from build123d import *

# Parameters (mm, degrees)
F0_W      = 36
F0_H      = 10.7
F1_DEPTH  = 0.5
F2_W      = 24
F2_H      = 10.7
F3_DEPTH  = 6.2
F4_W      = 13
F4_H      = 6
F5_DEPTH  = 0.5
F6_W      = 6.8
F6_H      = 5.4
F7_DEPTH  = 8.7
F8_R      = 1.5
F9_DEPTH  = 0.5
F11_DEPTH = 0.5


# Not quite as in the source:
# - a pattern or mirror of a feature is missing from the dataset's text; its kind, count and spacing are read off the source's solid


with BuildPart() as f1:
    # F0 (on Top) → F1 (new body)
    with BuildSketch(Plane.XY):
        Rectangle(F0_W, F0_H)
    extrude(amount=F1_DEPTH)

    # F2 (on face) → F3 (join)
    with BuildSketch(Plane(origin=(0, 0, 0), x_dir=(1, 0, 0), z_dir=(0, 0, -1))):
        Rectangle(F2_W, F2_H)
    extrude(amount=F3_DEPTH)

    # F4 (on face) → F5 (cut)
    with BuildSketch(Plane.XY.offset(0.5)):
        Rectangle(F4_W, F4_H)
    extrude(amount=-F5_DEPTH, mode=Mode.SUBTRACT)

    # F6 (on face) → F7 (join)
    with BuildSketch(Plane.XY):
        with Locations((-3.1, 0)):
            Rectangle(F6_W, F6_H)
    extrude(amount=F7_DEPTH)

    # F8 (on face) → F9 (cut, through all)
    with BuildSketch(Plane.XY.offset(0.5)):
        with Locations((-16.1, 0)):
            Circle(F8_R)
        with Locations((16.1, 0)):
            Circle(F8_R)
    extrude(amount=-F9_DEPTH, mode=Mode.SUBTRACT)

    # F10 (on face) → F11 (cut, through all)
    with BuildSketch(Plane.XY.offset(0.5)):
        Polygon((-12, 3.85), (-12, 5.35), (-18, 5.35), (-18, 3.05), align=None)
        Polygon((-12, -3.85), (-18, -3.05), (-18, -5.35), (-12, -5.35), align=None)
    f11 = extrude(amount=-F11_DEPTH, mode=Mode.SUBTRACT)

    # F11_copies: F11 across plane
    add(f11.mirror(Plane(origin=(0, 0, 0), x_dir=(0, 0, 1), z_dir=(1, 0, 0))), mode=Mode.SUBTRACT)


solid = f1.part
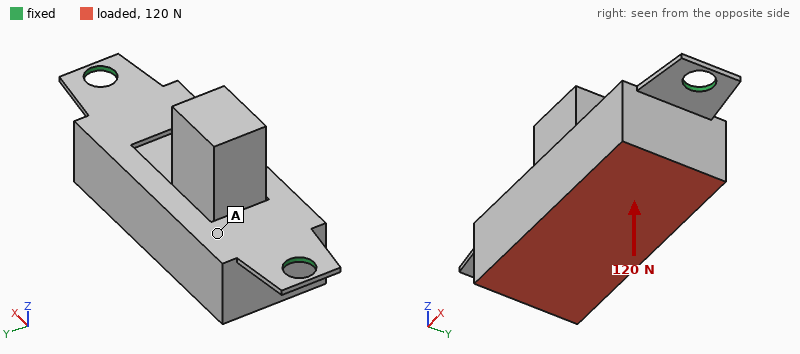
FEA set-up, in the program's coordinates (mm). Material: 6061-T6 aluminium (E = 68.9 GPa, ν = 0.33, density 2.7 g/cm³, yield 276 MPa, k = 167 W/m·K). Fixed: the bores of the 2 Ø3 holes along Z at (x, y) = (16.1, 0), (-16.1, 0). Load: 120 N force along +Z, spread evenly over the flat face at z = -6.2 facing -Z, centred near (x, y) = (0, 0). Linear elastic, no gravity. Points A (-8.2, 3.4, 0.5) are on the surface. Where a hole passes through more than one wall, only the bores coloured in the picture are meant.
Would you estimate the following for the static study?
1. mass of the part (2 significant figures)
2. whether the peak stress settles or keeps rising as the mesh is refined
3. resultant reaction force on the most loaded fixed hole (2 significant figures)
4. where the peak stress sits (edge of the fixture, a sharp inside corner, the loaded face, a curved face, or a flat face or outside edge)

5.5 g
keeps rising
76 N
edge of the fixture
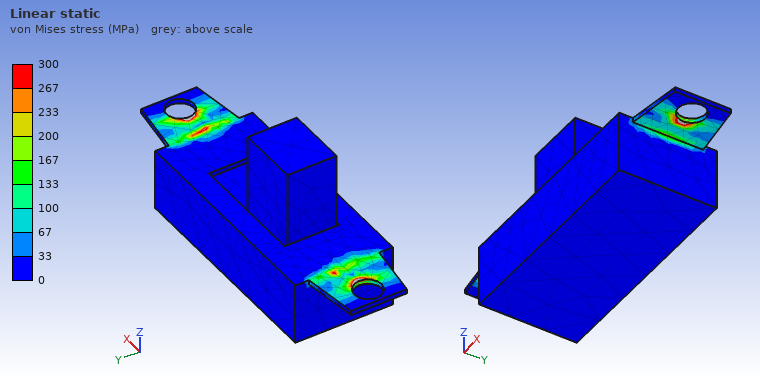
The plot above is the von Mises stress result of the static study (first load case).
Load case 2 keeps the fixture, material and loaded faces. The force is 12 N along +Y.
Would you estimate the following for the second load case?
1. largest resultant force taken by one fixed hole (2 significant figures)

6.0 N
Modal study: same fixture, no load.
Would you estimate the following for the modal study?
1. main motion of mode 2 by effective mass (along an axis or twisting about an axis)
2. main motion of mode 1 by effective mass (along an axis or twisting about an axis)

along Z
along Y
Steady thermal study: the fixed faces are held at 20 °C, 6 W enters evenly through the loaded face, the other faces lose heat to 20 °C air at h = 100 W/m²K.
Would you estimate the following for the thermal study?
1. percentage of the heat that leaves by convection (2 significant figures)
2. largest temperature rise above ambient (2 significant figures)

25 %
16 K
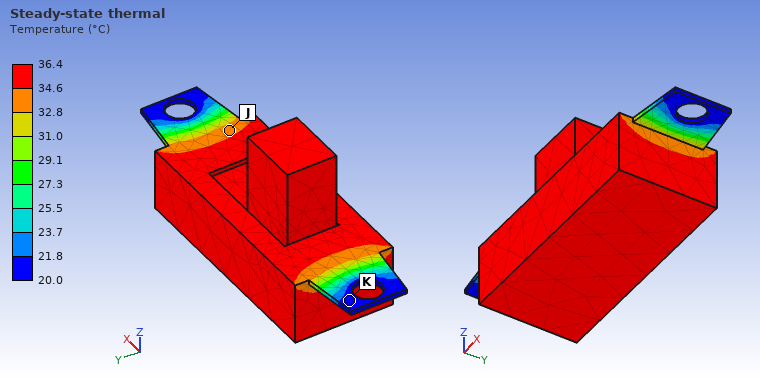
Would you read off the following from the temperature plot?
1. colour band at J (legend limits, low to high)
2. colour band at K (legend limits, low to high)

32.8 to 34.6 °C
20.0 to 21.8 °C
